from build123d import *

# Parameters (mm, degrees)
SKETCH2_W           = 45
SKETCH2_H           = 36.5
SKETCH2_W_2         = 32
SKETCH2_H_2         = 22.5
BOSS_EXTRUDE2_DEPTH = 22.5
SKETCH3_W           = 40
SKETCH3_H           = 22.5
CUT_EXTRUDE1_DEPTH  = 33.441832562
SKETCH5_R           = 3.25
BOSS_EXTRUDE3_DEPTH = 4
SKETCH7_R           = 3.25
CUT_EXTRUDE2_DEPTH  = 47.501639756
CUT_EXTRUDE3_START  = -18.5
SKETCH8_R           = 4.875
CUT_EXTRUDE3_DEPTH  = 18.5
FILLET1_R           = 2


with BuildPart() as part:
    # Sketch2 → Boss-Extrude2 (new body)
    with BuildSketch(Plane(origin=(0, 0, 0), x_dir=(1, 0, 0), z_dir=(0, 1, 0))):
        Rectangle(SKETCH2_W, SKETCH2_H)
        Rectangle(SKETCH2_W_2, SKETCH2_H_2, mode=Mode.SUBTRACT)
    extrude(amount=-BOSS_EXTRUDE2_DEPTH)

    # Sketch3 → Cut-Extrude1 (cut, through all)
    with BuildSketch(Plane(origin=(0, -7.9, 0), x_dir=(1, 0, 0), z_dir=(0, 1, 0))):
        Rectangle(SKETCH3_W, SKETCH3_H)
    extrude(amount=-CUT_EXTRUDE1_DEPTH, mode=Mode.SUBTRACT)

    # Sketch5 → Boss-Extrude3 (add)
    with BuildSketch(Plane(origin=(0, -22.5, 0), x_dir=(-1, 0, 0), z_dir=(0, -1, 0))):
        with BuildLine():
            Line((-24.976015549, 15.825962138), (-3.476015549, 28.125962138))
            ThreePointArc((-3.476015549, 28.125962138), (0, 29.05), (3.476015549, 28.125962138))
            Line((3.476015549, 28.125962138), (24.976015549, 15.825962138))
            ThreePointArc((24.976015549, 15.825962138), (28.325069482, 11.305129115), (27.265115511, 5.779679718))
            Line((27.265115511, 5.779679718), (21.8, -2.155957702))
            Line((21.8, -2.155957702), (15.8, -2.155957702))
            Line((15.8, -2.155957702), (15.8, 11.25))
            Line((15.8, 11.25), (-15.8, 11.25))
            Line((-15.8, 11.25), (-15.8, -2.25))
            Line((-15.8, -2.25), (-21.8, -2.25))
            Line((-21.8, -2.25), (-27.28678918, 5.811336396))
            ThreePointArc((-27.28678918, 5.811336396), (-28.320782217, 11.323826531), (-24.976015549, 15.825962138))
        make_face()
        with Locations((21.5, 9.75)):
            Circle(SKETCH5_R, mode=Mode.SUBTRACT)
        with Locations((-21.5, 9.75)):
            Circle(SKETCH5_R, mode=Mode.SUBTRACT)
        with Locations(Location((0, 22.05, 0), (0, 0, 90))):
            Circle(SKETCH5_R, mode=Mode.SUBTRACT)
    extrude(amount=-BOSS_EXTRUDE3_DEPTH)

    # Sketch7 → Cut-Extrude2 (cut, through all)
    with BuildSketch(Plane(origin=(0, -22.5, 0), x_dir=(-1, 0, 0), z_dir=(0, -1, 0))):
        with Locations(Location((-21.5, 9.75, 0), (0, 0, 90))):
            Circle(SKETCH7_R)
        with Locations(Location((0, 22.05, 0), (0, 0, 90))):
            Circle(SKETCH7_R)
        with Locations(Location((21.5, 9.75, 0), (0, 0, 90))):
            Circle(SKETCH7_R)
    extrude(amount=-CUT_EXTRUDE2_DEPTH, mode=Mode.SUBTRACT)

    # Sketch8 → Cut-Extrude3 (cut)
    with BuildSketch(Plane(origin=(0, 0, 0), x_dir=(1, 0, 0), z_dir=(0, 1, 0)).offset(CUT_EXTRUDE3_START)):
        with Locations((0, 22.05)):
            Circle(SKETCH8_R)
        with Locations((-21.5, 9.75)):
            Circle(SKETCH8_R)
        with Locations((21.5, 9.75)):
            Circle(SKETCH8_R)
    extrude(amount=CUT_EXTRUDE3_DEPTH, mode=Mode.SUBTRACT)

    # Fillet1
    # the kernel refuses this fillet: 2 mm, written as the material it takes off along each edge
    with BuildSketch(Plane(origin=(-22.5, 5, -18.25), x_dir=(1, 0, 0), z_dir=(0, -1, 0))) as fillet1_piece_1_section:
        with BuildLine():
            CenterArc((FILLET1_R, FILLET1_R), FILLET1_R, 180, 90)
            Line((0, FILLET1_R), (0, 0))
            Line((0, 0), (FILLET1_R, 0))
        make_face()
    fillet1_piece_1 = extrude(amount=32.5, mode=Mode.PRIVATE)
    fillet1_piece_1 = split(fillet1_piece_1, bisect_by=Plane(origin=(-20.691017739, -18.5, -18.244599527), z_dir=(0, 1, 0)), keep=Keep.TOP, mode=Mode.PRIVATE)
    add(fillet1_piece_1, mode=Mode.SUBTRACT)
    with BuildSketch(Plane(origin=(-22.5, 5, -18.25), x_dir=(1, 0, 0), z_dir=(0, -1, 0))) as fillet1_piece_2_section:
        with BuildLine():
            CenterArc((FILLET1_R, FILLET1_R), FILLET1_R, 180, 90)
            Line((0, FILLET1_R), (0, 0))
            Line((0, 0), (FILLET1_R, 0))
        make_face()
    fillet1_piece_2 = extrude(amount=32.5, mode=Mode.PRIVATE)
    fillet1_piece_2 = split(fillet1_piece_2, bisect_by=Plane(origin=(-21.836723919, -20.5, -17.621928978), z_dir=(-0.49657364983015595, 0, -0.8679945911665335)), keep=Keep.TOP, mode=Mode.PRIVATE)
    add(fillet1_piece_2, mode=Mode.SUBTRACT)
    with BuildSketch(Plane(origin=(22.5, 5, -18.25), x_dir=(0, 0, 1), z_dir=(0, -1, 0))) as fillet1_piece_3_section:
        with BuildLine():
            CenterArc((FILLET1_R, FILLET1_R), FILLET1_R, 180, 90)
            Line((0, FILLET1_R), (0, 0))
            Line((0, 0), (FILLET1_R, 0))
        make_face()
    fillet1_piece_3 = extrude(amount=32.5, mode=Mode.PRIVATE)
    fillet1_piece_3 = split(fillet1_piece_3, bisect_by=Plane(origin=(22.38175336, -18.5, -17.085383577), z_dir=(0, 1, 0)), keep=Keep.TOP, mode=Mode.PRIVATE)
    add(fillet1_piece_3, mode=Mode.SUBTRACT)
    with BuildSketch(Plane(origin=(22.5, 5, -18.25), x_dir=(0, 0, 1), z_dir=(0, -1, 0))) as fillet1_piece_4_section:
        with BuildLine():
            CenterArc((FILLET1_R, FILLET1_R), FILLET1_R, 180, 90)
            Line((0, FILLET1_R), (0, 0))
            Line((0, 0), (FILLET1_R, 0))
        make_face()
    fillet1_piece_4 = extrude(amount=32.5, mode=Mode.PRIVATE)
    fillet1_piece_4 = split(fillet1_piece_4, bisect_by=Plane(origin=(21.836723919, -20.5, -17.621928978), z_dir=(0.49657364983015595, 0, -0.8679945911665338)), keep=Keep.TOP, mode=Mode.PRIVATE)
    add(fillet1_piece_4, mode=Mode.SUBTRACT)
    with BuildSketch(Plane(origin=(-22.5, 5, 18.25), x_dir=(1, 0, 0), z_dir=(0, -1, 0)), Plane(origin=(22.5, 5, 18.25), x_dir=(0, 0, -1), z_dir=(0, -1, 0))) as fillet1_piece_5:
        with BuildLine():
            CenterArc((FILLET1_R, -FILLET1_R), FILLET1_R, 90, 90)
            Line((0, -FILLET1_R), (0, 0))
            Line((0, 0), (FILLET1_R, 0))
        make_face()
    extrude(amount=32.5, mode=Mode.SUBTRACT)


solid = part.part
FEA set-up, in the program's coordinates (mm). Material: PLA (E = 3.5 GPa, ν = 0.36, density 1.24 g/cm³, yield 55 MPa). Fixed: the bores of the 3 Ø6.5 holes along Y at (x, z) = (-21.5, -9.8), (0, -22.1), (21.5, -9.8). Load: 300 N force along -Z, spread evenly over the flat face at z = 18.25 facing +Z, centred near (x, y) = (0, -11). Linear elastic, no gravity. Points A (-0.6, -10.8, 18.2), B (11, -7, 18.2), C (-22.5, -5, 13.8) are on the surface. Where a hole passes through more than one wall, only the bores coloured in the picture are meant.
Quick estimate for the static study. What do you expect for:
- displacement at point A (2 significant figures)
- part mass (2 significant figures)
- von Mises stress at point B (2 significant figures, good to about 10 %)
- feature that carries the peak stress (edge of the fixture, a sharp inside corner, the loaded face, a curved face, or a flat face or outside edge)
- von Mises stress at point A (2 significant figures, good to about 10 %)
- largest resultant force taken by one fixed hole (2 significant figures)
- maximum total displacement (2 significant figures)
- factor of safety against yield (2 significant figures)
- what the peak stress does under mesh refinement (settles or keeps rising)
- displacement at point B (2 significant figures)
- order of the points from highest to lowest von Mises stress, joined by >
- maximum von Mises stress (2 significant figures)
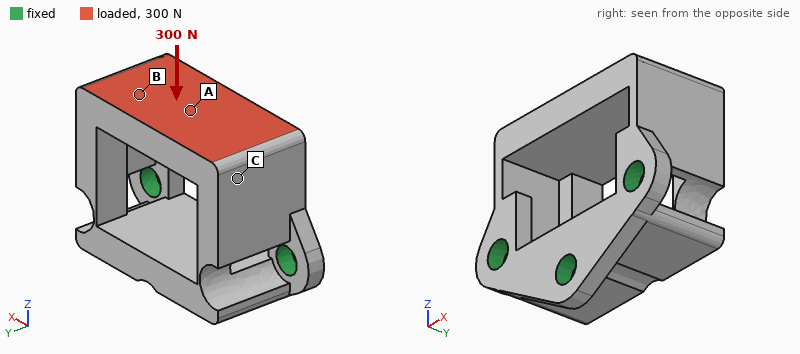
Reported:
0.24 mm
23 g
3.2 MPa
a curved face
5.5 MPa
150 N
0.30 mm
1.8
settles
0.24 mm
A > B > C
31 MPa
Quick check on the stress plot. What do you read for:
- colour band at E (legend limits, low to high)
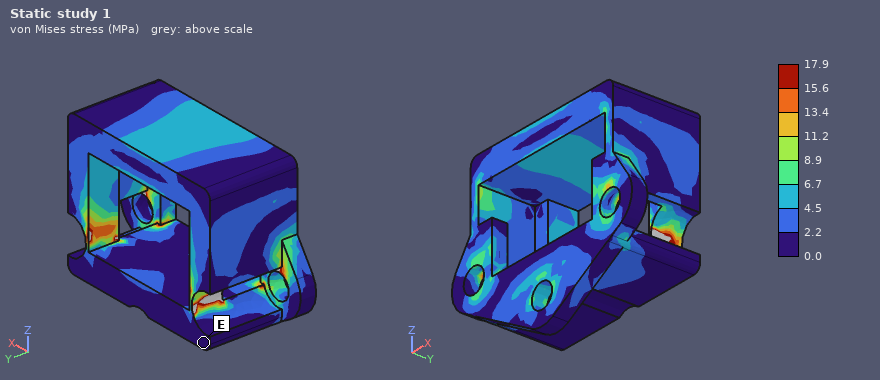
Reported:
0.0 to 2.2 MPa
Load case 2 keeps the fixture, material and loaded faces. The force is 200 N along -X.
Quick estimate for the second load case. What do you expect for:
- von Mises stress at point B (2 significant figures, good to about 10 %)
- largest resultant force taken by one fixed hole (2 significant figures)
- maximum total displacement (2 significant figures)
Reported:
3.4 MPa
130 N
0.36 mm
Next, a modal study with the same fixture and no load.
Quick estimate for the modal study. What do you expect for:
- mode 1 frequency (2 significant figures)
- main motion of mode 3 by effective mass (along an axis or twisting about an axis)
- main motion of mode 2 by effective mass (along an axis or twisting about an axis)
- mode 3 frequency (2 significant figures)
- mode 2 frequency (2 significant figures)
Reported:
1100 Hz
twisting about Z
along X
2400 Hz
1200 Hz
